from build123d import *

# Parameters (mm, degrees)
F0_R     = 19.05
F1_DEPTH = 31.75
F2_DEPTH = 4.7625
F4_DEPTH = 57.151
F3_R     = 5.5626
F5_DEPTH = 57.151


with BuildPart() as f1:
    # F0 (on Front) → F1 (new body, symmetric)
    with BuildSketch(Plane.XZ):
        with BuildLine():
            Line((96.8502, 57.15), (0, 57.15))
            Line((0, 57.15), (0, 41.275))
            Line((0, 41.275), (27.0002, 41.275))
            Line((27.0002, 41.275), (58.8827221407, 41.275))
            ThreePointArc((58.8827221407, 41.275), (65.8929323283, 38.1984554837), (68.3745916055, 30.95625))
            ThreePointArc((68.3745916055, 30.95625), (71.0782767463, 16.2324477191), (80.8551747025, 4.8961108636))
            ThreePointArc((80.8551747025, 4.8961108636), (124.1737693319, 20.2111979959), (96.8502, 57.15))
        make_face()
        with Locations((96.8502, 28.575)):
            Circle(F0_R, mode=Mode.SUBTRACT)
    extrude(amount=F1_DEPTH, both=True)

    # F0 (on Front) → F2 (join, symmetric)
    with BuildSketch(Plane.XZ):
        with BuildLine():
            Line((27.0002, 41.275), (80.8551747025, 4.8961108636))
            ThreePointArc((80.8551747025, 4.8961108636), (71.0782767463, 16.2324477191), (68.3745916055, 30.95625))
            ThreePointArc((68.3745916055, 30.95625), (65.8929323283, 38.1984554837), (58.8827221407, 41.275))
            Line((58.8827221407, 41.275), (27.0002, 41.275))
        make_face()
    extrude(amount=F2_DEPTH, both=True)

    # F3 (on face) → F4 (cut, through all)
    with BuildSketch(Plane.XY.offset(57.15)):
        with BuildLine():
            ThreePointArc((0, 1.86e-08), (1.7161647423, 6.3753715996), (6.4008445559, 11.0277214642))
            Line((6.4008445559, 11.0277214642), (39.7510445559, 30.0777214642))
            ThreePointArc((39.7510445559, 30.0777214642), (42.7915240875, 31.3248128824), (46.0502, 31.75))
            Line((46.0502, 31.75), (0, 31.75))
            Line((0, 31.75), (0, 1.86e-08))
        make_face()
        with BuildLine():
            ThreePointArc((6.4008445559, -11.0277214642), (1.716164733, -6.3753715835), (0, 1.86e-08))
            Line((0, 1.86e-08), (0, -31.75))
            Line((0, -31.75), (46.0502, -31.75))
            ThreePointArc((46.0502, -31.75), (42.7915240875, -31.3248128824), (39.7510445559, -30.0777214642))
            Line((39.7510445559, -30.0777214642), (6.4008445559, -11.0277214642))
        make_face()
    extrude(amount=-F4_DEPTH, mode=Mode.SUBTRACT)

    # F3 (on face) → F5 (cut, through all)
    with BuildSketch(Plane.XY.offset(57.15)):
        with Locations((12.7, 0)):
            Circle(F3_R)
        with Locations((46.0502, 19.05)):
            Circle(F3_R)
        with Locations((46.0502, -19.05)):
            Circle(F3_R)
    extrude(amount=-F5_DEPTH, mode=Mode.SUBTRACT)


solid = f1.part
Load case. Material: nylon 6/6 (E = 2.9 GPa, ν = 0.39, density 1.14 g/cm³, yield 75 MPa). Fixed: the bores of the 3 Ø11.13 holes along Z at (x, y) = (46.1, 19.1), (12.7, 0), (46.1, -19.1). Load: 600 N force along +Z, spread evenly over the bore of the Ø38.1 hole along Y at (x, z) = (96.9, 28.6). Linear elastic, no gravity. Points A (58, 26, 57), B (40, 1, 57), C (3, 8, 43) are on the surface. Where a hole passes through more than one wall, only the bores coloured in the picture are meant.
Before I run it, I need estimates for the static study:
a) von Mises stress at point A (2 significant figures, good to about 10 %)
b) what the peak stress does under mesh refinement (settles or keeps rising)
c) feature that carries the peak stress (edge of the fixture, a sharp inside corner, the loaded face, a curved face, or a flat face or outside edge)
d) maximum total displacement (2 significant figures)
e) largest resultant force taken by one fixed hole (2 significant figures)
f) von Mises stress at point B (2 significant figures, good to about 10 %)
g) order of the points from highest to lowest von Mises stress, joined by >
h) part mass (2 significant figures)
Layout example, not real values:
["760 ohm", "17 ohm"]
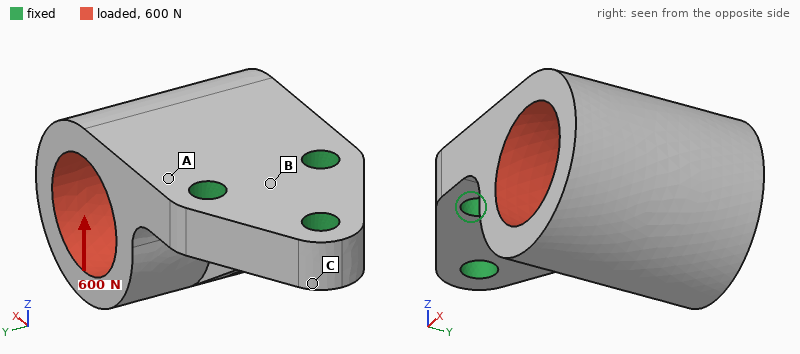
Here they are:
["5.5 MPa", "keeps rising", "edge of the fixture", "0.47 mm", "430 N", "2.5 MPa", "A > B > C", "180 g"]
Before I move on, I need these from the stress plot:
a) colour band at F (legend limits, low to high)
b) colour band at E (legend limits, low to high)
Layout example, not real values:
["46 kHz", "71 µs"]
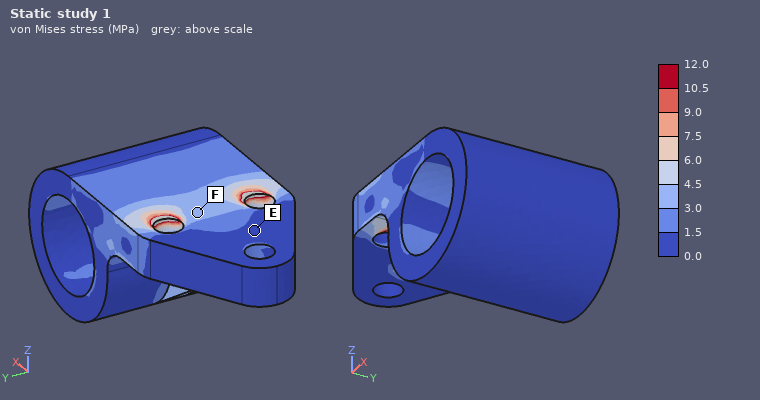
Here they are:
["3.0 to 4.5 MPa", "0.0 to 1.5 MPa"]
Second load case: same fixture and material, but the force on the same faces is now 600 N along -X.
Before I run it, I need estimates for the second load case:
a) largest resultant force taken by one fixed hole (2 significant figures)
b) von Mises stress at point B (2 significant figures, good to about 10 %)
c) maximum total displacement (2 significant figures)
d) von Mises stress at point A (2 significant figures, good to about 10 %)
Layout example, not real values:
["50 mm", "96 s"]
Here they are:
["240 N", "0.93 MPa", "0.22 mm", "1.9 MPa"]
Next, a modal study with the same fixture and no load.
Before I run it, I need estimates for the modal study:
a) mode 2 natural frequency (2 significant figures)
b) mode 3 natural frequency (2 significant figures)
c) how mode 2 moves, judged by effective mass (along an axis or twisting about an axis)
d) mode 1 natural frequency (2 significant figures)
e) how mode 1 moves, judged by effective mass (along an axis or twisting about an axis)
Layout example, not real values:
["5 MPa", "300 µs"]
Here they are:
["1100 Hz", "1800 Hz", "along Y", "600 Hz", "along Z"]
